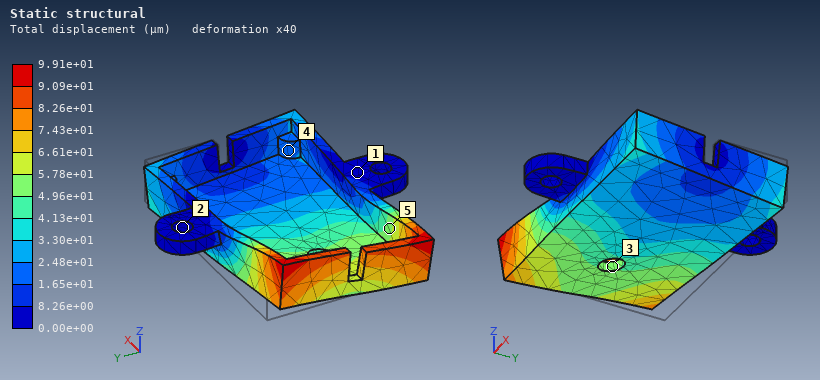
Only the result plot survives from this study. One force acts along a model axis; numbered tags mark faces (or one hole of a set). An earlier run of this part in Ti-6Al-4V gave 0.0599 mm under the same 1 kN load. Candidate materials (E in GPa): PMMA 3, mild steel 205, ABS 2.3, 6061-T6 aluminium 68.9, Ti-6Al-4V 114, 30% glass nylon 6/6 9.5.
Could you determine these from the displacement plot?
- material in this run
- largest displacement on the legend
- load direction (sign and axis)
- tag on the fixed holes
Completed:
6061-T6 aluminium
9.91e+01 µm
-Y
2
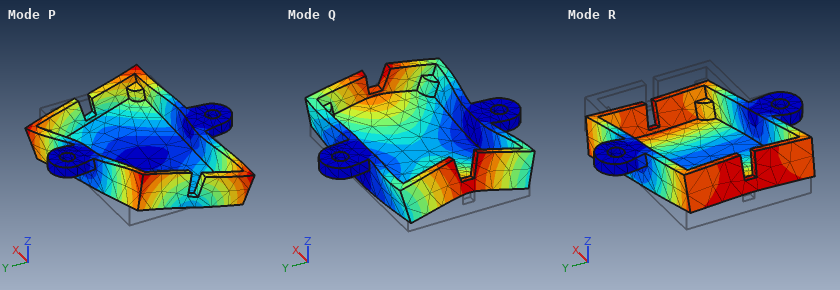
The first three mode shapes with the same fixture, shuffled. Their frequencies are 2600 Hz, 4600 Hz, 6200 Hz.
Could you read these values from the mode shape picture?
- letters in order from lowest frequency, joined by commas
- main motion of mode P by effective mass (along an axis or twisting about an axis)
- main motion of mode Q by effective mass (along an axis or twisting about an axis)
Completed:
R, P, Q
twisting about Z
along Z
